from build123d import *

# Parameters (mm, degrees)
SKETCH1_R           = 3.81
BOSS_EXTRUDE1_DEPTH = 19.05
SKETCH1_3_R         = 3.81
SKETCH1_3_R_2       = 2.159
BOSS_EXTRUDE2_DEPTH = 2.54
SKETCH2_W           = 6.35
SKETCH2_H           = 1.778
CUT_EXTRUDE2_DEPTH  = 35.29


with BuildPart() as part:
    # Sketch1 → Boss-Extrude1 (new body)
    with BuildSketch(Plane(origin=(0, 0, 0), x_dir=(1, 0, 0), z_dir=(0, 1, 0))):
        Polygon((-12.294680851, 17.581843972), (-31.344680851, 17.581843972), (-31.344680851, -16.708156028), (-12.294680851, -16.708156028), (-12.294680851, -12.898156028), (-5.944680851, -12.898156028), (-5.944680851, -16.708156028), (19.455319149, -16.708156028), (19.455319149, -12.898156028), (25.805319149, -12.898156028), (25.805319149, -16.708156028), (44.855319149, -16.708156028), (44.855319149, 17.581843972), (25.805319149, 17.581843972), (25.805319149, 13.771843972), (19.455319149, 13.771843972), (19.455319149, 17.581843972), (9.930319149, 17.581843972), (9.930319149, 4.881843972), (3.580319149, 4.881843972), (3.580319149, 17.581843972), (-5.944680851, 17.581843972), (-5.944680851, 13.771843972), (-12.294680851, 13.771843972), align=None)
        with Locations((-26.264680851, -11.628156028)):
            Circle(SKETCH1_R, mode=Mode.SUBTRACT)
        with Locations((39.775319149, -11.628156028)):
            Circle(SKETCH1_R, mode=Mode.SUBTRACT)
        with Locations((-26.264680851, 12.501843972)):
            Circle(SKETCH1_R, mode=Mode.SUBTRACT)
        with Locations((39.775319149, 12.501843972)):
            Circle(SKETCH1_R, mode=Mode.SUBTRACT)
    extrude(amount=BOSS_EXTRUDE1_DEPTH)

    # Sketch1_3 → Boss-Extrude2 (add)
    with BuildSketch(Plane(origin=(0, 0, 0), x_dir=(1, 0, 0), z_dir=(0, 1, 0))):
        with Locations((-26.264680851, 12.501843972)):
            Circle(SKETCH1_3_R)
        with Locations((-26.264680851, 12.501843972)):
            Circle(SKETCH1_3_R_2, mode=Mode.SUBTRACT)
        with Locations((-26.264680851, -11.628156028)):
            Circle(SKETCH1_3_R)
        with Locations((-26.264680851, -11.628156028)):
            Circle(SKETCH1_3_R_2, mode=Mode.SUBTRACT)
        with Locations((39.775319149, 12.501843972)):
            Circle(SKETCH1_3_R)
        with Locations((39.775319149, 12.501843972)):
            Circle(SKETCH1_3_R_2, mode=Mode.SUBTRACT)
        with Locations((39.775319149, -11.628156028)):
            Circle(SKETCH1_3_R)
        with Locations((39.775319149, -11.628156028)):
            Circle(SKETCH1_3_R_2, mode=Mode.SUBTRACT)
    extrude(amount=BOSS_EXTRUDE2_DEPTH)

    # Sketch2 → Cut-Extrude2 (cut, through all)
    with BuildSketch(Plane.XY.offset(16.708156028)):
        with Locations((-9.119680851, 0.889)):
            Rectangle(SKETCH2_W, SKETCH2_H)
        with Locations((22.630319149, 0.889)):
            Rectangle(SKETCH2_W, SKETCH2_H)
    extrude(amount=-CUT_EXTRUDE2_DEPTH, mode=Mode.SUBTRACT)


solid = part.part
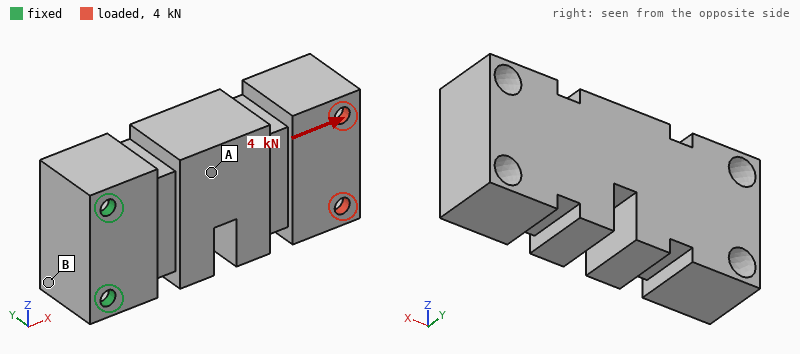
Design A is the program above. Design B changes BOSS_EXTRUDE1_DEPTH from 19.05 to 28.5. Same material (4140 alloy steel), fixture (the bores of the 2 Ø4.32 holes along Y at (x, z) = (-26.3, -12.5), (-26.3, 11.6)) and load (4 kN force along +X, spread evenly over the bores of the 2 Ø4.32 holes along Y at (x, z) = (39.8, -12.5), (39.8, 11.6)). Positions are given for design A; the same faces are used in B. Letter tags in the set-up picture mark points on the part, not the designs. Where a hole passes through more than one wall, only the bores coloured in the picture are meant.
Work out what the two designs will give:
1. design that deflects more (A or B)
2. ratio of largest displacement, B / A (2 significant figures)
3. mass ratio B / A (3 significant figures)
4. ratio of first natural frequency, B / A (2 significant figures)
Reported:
A
0.58
1.50
0.81
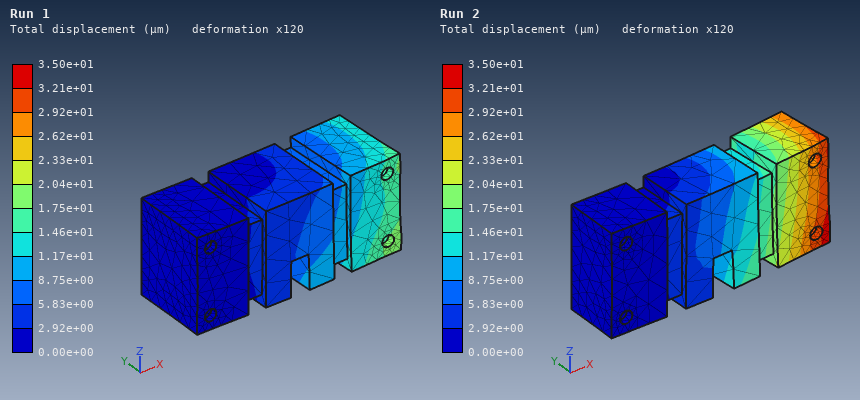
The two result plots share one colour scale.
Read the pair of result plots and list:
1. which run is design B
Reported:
Run 1
